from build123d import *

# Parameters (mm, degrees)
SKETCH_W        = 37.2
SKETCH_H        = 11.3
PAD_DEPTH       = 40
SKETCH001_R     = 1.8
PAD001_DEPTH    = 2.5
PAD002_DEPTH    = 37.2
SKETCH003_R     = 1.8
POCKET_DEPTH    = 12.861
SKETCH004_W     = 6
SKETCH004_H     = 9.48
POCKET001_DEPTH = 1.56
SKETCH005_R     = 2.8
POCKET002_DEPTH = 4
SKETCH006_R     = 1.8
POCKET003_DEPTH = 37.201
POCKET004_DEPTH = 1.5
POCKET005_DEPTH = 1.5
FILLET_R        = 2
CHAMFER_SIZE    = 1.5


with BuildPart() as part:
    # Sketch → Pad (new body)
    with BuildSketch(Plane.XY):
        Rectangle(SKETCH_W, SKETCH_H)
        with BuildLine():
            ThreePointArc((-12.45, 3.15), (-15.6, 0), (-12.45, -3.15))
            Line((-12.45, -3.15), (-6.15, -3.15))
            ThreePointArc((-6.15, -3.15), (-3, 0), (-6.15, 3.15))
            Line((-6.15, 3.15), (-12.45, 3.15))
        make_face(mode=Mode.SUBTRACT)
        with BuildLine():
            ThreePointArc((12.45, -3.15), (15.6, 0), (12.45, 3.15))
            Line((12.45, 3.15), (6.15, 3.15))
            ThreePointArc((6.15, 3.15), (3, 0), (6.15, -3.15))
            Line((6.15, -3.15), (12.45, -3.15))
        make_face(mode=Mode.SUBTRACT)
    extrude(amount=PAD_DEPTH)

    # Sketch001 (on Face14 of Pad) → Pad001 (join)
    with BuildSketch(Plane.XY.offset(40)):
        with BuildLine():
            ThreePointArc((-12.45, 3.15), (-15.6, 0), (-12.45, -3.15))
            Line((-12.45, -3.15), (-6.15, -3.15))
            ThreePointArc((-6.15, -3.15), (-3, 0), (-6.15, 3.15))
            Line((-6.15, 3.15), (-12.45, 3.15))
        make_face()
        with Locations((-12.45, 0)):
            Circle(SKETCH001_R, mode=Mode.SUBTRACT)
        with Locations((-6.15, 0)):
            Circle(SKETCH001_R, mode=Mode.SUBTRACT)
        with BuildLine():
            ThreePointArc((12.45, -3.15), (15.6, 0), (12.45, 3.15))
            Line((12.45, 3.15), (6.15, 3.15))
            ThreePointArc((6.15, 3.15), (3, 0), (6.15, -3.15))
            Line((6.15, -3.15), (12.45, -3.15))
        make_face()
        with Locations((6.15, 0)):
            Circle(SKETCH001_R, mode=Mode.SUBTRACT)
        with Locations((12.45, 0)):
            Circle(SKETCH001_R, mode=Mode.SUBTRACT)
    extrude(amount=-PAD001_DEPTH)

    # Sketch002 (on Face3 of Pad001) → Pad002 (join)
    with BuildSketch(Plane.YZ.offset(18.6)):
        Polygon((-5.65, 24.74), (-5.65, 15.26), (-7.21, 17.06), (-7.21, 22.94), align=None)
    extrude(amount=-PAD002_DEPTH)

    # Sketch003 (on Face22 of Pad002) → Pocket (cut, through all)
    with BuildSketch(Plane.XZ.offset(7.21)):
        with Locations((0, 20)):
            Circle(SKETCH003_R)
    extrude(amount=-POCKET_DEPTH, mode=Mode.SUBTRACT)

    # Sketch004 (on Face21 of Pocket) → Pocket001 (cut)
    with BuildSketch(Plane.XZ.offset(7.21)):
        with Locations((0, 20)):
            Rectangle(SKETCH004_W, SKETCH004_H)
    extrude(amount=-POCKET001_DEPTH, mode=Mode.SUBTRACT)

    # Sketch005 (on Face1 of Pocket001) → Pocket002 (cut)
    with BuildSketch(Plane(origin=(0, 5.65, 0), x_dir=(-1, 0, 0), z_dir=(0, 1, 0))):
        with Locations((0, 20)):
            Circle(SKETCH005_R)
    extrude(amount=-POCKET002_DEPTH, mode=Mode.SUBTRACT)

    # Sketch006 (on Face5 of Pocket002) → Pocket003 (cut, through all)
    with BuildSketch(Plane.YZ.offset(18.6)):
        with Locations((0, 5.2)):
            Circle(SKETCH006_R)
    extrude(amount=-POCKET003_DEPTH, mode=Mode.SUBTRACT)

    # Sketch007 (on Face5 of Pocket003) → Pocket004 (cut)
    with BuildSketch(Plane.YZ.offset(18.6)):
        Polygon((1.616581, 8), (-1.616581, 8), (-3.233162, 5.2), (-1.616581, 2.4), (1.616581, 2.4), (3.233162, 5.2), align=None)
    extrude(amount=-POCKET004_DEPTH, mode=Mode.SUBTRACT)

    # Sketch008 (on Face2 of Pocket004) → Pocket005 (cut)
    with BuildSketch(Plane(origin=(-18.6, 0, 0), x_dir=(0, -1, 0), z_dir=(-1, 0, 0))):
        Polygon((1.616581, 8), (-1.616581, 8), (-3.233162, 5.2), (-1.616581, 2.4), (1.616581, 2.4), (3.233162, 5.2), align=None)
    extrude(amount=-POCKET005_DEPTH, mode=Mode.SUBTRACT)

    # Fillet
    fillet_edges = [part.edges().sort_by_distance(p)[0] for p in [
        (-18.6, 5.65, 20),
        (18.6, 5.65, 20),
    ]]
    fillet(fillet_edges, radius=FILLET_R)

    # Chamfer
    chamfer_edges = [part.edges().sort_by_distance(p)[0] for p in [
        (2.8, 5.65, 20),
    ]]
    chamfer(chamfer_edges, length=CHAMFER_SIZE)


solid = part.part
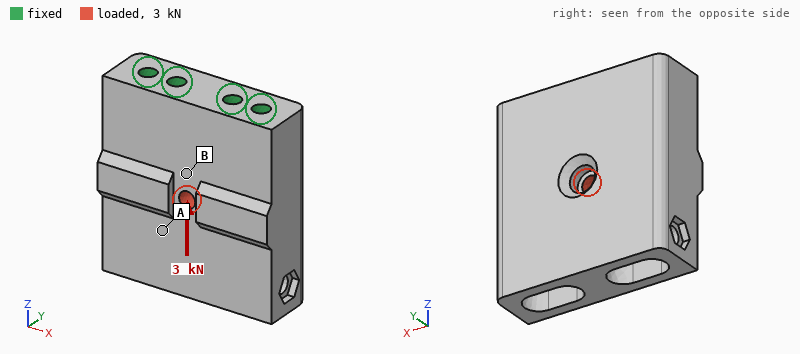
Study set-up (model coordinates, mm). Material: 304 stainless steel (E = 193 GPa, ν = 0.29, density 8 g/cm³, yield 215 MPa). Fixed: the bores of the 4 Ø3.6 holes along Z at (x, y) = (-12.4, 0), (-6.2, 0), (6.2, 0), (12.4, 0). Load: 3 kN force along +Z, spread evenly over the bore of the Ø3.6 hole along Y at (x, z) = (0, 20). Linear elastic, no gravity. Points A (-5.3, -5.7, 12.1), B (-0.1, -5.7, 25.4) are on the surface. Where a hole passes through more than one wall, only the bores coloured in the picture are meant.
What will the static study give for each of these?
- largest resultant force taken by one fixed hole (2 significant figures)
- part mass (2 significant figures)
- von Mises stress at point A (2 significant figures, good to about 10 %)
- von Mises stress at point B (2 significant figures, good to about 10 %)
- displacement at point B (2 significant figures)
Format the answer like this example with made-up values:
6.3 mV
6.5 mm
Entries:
860 N
91 g
13 MPa
32 MPa
7.1 µm
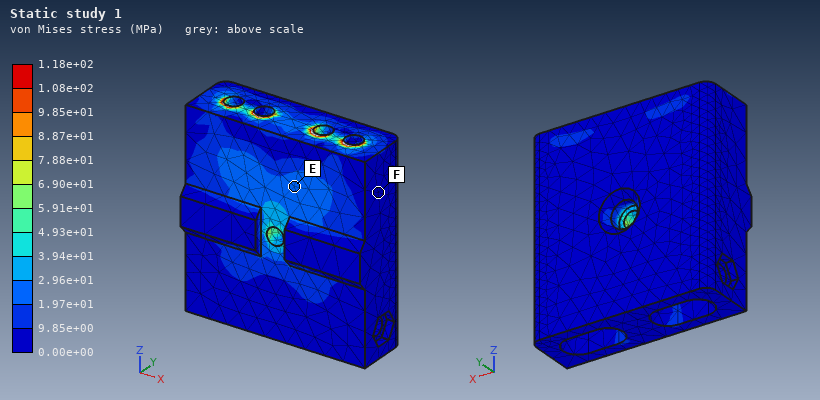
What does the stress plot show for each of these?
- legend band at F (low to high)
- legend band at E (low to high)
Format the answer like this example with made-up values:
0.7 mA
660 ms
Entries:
0.00e+00 to 9.85e+00 MPa
1.97e+01 to 2.96e+01 MPa
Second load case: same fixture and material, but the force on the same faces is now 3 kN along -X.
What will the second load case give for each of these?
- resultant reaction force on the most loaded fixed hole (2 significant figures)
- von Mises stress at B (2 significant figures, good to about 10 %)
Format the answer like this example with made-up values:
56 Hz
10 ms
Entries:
1.8 kN
36 MPa
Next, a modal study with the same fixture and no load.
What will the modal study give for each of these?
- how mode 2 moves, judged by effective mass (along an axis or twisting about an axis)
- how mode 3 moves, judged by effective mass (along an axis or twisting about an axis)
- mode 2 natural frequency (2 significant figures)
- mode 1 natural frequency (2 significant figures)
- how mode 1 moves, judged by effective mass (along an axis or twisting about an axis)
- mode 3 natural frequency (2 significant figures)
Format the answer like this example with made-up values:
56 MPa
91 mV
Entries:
along X
twisting about Z
8300 Hz
2900 Hz
along Y
10 kHz
